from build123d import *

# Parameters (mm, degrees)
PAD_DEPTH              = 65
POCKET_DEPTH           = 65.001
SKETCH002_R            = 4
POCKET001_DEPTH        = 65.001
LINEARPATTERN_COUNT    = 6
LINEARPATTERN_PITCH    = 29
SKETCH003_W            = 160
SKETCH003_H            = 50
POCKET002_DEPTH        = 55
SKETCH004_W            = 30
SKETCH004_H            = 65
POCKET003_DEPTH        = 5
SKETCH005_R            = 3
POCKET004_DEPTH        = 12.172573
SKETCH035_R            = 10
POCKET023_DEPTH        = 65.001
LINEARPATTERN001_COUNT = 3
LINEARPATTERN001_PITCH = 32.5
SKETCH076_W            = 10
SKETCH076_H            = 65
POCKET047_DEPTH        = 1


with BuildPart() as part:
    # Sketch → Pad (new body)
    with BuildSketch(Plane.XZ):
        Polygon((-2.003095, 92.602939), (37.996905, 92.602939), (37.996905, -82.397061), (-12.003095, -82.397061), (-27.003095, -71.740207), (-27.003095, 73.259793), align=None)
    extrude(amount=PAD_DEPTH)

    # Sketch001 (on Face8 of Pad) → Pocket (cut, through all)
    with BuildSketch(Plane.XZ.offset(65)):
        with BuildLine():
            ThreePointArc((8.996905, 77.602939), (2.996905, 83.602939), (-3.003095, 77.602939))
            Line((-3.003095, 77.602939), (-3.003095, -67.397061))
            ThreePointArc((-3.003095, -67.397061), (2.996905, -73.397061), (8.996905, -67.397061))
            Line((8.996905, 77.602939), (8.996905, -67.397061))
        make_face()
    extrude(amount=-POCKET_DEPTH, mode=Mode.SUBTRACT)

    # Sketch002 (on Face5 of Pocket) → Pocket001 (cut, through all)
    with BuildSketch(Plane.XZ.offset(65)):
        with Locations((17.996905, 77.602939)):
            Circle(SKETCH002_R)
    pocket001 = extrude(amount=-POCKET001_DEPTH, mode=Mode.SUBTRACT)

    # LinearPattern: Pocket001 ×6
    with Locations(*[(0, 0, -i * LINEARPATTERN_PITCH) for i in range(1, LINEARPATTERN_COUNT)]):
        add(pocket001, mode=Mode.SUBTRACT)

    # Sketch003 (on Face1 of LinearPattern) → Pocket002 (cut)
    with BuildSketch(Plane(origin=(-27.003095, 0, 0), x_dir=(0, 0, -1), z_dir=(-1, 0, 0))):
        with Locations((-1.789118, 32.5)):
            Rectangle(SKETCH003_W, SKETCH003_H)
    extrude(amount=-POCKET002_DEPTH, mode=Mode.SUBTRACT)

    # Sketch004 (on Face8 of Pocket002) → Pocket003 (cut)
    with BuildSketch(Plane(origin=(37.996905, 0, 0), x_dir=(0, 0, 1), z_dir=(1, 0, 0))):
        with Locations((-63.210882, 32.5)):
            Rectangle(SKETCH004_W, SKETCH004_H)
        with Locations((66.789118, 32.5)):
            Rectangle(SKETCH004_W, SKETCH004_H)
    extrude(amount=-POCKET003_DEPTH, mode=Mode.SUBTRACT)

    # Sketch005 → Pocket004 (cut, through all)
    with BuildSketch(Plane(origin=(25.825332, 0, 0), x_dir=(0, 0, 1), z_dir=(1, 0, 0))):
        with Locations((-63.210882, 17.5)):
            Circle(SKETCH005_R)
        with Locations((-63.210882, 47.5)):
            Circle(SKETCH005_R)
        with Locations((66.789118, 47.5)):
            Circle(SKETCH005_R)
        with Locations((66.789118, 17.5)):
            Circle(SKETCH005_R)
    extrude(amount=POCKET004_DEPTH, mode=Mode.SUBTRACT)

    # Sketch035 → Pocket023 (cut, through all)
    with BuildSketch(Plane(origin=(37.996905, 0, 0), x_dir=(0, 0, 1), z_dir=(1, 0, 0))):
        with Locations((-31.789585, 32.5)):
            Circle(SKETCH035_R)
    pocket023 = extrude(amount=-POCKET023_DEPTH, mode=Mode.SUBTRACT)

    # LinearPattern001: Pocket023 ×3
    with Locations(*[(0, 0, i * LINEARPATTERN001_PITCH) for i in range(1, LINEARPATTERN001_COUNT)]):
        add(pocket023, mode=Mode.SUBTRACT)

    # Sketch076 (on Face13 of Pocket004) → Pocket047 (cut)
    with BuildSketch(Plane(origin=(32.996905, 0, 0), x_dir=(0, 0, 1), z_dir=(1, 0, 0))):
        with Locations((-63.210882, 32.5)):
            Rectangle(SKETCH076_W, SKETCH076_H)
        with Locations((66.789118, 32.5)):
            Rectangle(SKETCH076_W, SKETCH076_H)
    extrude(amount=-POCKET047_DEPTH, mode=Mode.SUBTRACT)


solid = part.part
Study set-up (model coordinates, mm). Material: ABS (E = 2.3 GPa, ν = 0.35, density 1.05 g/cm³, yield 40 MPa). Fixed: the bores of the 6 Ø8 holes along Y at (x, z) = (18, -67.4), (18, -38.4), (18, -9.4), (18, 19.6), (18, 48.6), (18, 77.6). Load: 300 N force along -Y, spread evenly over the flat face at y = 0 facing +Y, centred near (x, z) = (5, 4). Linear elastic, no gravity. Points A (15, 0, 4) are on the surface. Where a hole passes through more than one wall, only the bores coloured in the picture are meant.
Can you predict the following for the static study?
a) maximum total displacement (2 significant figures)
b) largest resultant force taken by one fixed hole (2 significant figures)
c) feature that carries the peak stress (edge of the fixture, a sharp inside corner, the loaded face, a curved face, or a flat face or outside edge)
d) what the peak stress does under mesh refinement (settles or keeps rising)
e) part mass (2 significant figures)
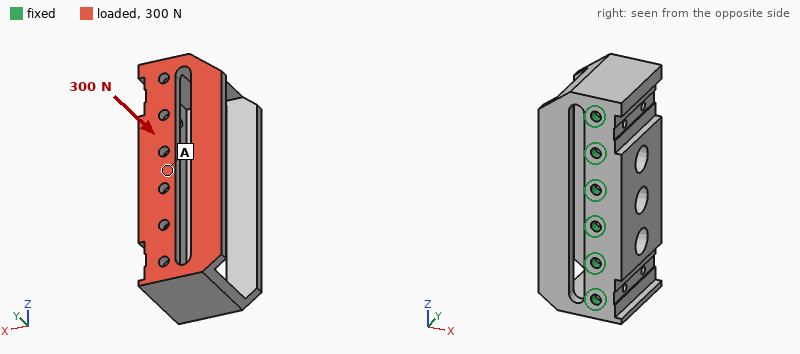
2.0 mm
150 N
edge of the fixture
keeps rising
230 g
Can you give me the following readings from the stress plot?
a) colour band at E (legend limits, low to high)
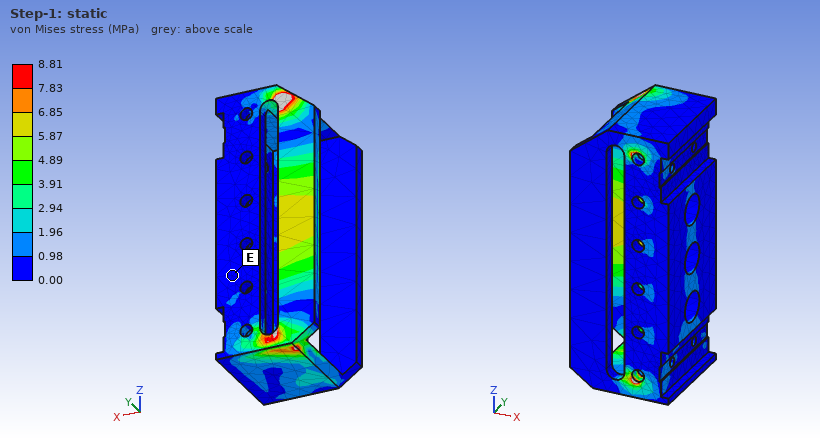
0.00 to 0.98 MPa
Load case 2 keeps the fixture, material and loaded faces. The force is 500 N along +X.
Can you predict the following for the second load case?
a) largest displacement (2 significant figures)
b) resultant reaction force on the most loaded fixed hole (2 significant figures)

2.0 mm
340 N
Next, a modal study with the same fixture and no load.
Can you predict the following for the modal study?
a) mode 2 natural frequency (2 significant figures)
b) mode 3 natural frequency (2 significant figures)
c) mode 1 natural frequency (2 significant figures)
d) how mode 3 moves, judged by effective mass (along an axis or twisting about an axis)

290 Hz
370 Hz
260 Hz
along X
